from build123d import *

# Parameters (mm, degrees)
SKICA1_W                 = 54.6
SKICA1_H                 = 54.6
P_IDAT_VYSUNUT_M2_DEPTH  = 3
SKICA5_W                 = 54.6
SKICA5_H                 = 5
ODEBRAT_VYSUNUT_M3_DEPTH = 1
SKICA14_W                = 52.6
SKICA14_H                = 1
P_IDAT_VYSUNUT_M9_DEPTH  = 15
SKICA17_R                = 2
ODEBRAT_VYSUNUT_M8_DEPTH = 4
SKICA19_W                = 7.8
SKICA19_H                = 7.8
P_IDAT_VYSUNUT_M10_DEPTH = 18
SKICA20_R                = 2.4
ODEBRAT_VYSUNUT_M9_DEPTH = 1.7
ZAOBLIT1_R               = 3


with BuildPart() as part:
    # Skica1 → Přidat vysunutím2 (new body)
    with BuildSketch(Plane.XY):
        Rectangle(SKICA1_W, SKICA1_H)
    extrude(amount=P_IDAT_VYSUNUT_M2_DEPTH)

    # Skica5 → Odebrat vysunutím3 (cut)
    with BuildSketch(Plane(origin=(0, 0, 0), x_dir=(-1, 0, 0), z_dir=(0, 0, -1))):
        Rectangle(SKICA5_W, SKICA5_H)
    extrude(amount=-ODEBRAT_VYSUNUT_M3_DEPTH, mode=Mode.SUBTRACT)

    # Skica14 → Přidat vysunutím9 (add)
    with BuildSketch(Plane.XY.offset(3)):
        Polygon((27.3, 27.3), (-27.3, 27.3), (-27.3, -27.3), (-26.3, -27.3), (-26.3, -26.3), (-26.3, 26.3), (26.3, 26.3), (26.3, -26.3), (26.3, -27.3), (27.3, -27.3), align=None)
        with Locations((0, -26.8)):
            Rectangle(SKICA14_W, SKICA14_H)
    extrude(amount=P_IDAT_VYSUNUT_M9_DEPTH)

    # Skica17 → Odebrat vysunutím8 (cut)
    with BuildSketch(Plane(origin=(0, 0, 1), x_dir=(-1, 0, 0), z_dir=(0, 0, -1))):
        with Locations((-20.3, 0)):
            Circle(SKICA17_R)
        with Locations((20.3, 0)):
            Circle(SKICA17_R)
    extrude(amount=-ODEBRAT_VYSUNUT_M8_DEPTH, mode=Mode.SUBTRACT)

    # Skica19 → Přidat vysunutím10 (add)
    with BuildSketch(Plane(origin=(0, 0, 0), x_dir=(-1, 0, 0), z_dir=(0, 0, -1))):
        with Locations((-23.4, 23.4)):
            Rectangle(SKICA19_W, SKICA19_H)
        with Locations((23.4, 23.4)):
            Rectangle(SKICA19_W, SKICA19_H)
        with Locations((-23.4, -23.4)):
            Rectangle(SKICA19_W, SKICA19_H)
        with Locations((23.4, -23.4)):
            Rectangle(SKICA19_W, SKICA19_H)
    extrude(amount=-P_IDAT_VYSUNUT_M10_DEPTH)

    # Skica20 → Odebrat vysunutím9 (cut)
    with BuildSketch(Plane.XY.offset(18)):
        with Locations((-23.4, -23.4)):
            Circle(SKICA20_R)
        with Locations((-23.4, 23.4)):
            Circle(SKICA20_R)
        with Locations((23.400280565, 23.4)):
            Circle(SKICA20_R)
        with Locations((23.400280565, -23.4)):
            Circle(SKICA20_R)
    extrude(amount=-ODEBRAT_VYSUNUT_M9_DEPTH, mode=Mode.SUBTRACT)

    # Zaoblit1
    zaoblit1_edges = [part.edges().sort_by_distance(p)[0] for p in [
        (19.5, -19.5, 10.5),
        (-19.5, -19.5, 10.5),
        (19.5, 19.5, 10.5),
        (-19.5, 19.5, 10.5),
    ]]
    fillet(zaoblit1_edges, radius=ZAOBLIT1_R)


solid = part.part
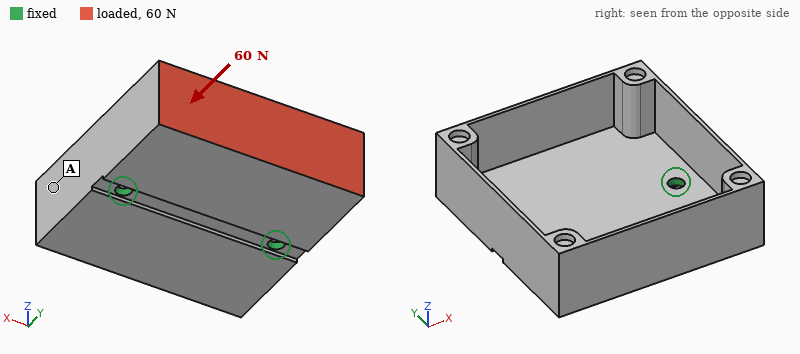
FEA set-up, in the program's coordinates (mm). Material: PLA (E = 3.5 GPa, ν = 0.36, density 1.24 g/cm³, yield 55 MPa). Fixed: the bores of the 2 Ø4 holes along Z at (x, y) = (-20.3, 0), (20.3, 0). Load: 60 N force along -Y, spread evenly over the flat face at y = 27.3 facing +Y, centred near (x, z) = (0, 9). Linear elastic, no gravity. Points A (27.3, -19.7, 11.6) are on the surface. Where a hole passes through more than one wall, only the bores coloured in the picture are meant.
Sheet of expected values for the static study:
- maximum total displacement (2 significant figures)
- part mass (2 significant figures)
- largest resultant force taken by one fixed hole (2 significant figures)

0.78 mm
18 g
31 N
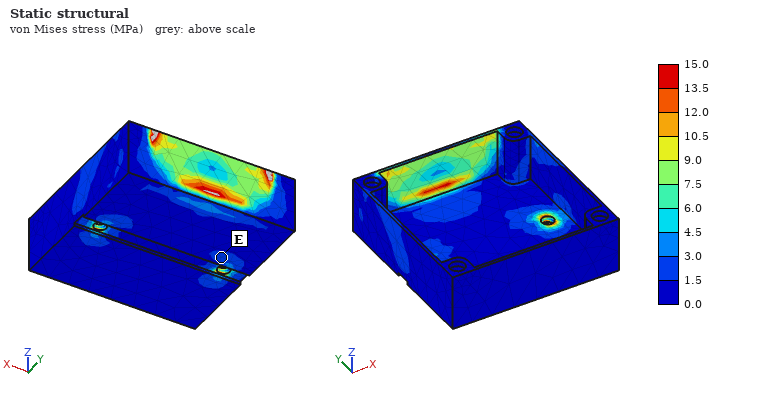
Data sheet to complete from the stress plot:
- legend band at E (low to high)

1.5 to 3.0 MPa
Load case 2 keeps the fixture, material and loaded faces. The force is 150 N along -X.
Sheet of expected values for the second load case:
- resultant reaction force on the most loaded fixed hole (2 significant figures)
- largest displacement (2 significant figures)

120 N
0.53 mm
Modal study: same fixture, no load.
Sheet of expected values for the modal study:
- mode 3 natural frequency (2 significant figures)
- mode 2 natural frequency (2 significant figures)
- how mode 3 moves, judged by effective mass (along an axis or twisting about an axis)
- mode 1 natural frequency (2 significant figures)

1500 Hz
760 Hz
along Z
510 Hz
